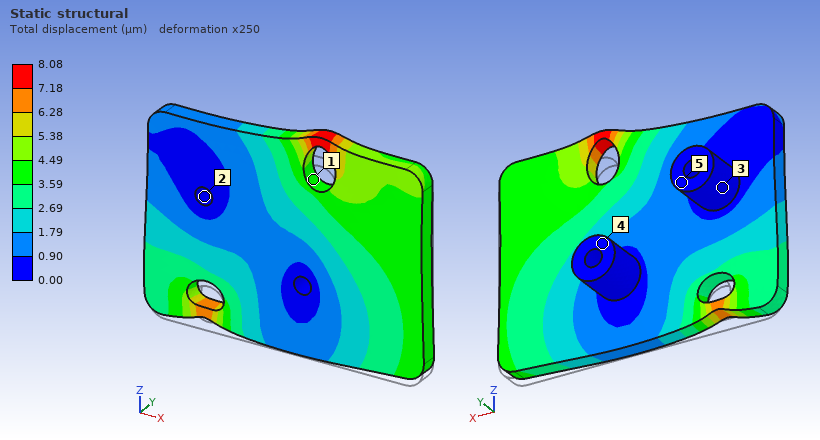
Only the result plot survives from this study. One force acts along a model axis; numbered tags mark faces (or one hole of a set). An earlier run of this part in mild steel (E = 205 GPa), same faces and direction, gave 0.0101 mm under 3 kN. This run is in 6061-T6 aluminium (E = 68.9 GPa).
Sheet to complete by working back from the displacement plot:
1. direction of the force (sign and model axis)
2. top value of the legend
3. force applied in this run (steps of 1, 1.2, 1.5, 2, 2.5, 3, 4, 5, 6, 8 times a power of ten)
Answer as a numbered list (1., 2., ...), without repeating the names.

1. +Z
2. 8.08 µm
3. 800 N
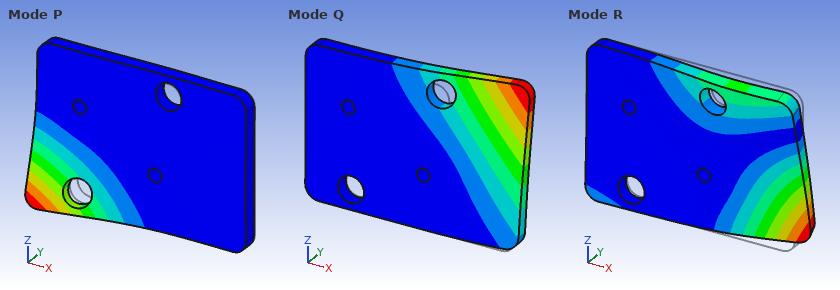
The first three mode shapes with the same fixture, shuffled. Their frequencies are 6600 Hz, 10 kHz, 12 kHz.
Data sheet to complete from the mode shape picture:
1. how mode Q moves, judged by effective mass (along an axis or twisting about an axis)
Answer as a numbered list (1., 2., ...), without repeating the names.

1. along Y
